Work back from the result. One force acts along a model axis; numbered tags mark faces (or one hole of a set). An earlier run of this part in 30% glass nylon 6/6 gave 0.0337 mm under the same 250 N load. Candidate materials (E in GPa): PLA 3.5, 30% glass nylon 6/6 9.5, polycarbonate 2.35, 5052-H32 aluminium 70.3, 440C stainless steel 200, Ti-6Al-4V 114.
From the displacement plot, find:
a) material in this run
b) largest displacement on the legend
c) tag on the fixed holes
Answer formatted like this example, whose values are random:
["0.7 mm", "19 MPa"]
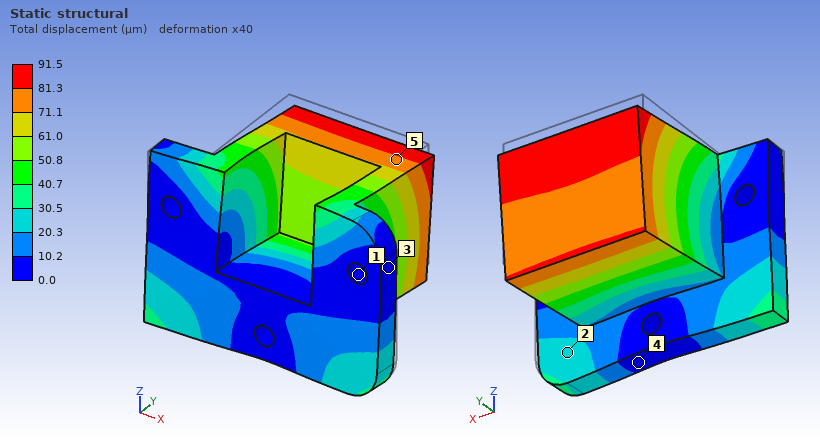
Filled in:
["PLA", "91.5 µm", "1"]
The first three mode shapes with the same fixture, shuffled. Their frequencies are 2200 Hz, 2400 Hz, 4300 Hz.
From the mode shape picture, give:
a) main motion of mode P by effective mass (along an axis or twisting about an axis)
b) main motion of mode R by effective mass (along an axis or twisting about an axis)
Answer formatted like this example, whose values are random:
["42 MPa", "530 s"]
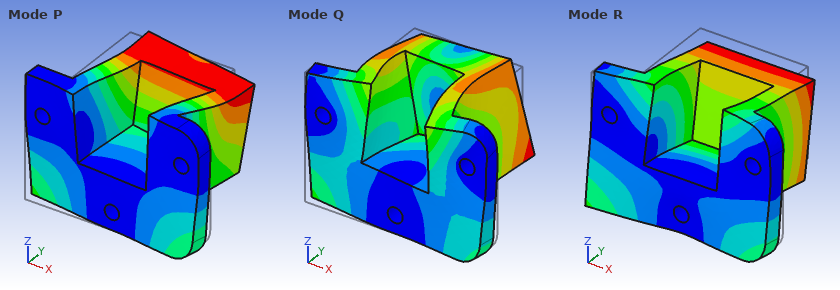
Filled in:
["along X", "along Z"]
